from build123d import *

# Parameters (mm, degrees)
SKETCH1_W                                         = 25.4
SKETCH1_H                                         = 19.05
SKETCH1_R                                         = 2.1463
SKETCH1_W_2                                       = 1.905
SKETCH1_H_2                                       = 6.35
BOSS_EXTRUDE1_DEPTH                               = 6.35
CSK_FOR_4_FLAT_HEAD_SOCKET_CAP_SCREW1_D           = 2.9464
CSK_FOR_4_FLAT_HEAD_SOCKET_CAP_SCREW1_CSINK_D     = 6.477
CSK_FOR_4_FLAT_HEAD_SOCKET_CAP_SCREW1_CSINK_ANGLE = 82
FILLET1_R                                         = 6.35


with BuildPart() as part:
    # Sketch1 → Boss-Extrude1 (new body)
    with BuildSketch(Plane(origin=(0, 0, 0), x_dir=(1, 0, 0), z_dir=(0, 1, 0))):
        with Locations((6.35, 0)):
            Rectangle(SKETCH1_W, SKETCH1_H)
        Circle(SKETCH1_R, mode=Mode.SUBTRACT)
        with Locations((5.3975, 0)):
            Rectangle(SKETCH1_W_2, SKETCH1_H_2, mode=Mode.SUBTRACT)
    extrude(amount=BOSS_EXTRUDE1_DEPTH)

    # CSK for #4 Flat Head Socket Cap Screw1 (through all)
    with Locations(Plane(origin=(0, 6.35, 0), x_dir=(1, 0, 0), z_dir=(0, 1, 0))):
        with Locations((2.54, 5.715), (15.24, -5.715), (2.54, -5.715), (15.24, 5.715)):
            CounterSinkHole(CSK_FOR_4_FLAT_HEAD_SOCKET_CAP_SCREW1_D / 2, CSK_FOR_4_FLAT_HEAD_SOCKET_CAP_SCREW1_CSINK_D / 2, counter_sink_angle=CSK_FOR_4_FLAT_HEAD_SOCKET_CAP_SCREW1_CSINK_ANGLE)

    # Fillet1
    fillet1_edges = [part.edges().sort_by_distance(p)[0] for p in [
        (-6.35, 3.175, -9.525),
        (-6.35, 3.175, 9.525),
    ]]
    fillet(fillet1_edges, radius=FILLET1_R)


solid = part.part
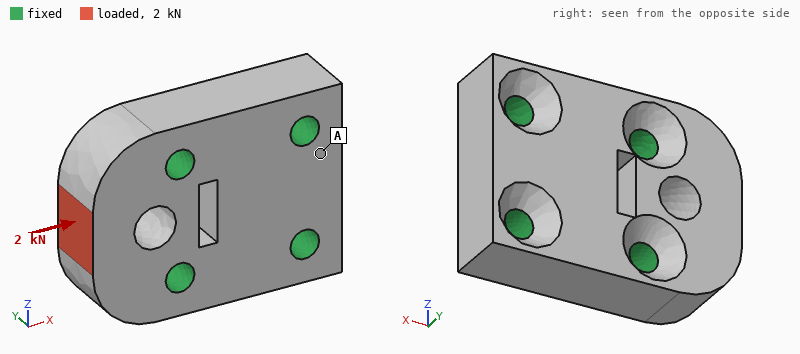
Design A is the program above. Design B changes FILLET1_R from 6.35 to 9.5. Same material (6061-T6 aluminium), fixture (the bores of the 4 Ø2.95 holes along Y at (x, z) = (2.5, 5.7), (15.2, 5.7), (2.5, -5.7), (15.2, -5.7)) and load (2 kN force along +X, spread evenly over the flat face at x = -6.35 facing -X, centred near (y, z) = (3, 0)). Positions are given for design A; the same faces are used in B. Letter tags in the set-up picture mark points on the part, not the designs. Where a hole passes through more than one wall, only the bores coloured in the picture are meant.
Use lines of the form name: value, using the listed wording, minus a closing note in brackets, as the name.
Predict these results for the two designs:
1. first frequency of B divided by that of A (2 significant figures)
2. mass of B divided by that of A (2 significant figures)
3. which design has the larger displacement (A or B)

first frequency of B divided by that of A: 1.1
mass of B divided by that of A: 0.95
which design has the larger displacement: B
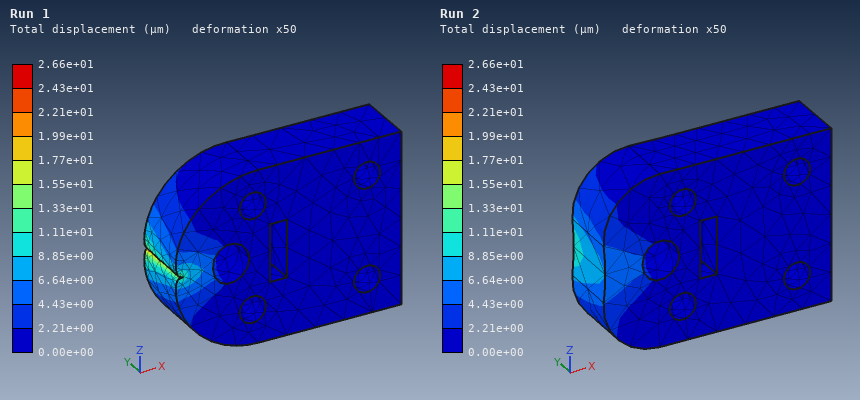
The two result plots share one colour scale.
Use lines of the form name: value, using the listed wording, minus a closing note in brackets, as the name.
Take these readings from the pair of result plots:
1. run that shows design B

run that shows design B: Run 1
